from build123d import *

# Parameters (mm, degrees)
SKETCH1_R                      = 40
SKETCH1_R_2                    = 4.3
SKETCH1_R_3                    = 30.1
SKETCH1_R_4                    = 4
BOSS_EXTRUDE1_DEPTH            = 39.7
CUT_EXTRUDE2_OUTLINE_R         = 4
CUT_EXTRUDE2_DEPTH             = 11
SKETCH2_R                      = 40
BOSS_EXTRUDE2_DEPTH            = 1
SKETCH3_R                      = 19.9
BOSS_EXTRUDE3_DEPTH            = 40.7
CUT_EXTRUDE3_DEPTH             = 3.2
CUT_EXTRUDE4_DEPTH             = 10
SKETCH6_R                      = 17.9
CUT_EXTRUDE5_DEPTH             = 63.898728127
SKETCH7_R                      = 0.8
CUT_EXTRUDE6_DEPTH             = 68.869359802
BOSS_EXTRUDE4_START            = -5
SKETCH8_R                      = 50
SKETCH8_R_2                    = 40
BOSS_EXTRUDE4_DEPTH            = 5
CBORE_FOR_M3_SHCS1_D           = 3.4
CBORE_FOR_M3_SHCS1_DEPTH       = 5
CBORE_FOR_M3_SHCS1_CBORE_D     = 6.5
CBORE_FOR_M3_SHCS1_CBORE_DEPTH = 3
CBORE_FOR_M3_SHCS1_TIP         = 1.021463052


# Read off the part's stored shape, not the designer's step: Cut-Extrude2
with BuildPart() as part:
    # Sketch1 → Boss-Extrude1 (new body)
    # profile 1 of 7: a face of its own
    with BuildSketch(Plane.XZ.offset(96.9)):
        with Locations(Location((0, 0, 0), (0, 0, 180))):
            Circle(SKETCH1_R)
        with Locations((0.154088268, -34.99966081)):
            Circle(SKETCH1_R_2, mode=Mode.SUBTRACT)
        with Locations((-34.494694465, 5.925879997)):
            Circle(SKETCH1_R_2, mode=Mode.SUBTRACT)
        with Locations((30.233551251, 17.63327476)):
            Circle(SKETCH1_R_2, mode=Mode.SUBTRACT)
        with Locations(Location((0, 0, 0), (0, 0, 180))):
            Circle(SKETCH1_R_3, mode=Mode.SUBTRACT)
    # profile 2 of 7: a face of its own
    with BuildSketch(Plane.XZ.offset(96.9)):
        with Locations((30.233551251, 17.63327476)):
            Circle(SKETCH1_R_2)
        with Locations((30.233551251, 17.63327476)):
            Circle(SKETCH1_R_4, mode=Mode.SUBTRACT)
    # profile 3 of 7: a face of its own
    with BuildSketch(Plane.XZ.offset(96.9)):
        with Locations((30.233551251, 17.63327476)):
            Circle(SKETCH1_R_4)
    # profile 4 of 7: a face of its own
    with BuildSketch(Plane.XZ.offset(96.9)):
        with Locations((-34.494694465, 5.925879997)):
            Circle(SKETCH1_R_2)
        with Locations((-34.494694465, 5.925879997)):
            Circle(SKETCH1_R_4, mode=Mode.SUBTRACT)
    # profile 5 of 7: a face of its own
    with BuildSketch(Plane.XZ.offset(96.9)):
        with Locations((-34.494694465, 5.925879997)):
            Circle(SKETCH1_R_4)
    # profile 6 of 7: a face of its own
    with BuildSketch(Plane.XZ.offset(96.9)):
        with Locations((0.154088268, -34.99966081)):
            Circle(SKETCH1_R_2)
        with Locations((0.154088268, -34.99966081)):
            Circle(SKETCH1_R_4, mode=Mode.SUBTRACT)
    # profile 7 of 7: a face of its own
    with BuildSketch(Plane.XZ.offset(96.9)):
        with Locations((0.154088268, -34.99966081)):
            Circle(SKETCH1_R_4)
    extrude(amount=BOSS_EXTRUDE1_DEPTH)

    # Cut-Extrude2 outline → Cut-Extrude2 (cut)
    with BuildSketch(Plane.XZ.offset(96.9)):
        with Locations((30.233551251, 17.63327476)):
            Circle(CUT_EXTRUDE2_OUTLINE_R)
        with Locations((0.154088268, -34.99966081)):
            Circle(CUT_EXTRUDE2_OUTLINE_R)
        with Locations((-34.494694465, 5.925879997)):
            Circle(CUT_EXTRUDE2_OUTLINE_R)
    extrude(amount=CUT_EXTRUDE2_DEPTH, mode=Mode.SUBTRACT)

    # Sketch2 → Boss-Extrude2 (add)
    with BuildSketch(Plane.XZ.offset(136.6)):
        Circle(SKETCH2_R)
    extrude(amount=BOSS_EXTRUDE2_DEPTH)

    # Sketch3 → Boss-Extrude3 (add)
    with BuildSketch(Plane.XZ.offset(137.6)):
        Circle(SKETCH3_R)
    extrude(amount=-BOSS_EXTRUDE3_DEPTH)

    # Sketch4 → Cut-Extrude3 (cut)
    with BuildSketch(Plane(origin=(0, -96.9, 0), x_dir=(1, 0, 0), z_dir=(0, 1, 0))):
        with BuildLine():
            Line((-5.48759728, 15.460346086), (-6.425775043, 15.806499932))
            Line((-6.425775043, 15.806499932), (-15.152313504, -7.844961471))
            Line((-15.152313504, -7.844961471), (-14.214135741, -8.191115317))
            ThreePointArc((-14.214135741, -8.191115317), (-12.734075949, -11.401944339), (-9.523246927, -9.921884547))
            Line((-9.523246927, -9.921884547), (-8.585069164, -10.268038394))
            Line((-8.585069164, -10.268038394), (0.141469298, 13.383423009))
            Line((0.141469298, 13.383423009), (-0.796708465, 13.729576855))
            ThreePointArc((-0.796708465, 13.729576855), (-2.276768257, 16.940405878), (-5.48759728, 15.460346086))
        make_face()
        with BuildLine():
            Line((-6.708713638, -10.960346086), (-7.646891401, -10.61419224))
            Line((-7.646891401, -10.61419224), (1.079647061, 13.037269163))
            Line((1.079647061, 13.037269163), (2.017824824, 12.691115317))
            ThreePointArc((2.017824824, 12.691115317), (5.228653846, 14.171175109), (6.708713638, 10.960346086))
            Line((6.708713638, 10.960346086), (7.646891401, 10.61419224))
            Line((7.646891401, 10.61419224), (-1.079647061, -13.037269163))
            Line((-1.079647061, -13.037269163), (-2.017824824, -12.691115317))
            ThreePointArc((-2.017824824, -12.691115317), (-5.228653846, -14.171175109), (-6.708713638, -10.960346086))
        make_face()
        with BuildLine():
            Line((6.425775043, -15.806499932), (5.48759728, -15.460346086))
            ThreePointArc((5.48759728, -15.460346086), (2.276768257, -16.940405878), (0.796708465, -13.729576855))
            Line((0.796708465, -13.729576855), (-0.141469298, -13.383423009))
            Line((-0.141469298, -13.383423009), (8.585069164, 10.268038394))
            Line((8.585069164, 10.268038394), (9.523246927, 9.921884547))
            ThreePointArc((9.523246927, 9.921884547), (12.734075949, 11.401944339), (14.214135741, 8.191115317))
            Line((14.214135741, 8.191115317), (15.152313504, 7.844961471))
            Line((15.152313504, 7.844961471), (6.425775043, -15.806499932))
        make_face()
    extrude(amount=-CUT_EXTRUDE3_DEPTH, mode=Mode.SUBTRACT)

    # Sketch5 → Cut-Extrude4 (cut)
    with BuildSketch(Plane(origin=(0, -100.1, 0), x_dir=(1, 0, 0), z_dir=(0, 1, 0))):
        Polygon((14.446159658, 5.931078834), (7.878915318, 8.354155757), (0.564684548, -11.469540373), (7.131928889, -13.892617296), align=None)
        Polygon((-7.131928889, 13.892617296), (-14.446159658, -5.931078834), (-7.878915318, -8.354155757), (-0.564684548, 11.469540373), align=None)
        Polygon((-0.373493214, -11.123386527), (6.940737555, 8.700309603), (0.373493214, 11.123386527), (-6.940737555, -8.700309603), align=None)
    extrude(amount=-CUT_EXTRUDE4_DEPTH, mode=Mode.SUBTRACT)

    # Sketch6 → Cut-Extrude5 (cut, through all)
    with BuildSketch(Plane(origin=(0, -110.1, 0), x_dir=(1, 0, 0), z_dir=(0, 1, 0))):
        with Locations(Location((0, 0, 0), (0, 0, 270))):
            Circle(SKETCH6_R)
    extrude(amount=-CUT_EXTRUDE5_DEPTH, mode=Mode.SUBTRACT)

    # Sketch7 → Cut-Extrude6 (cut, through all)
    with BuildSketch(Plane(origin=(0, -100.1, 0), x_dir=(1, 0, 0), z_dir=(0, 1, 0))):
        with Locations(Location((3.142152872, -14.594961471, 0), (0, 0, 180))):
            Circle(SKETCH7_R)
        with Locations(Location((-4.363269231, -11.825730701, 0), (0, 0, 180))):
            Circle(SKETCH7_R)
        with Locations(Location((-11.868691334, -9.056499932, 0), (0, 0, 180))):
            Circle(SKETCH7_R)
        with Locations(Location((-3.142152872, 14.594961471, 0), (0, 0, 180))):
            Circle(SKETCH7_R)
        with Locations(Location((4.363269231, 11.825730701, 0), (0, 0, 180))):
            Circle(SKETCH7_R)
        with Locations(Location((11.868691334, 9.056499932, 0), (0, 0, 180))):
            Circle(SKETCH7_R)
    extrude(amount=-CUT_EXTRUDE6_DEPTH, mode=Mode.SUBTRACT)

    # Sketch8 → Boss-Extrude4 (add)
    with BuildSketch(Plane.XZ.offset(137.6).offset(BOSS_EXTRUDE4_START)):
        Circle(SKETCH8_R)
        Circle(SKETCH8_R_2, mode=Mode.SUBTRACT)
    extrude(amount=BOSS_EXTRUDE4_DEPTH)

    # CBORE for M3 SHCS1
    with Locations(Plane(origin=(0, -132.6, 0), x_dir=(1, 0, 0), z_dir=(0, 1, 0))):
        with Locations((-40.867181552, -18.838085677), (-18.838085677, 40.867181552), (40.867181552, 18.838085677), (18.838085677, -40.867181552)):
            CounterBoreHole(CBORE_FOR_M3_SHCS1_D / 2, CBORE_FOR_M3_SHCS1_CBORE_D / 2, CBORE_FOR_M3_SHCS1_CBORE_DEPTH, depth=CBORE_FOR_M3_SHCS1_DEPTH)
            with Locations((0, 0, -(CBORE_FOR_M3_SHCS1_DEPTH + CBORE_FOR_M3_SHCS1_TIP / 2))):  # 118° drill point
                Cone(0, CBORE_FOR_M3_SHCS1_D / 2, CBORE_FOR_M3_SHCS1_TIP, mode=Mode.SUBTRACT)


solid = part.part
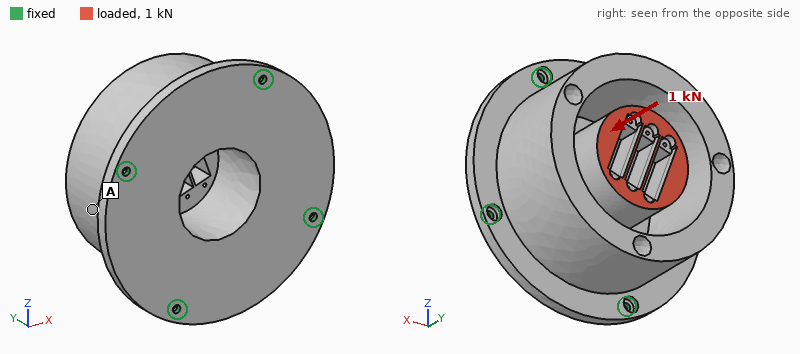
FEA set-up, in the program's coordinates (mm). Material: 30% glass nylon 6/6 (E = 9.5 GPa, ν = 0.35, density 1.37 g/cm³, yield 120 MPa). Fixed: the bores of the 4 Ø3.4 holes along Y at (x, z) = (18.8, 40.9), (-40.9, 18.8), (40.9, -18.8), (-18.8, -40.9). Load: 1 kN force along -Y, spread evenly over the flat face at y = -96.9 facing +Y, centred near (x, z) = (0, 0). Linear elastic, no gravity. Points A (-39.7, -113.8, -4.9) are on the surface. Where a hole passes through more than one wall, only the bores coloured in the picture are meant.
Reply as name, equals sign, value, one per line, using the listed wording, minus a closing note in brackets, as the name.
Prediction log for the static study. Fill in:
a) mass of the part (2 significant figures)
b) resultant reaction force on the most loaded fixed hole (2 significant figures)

mass of the part = 160 g
resultant reaction force on the most loaded fixed hole = 350 N
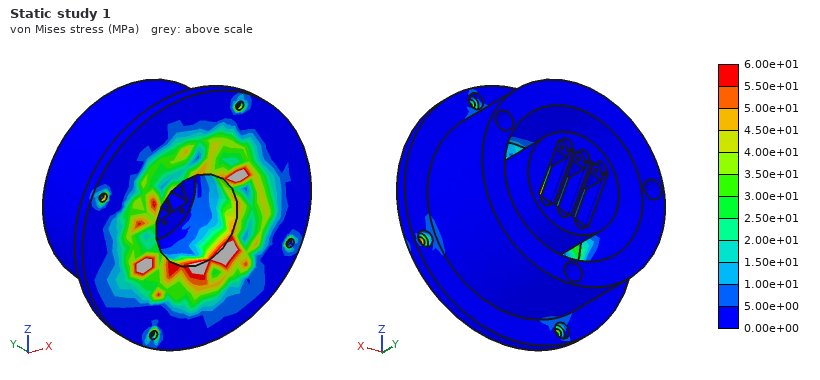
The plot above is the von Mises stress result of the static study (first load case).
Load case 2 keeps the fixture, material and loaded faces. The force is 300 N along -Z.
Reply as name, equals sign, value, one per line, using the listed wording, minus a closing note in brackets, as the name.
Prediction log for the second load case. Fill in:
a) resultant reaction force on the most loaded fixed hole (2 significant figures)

resultant reaction force on the most loaded fixed hole = 190 N
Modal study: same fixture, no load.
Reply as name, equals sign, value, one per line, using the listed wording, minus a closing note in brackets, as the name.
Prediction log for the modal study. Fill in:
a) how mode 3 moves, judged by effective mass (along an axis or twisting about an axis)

how mode 3 moves, judged by effective mass = along Y
